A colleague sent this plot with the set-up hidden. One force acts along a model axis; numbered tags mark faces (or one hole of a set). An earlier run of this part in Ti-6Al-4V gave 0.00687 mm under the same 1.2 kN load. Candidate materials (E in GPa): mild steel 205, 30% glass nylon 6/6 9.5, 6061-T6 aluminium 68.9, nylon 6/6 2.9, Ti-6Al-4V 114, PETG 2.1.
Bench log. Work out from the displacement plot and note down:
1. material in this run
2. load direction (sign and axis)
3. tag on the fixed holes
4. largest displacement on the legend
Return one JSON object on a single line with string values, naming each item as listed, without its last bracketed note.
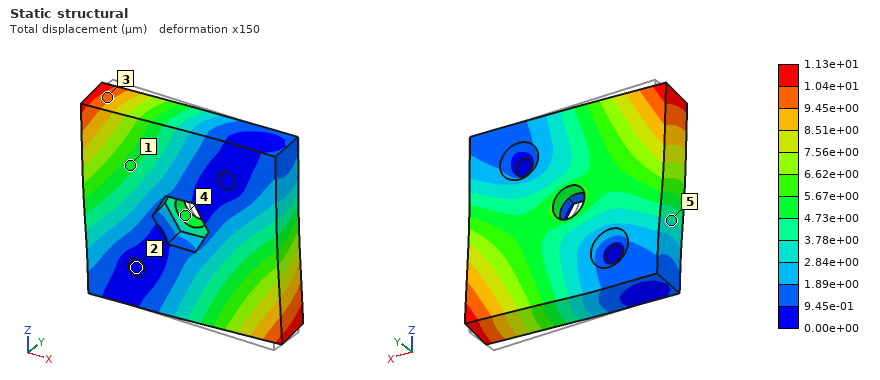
{"material in this run": "6061-T6 aluminium", "load direction": "-X", "tag on the fixed holes": "2", "largest displacement on the legend": "1.13e+01 µm"}
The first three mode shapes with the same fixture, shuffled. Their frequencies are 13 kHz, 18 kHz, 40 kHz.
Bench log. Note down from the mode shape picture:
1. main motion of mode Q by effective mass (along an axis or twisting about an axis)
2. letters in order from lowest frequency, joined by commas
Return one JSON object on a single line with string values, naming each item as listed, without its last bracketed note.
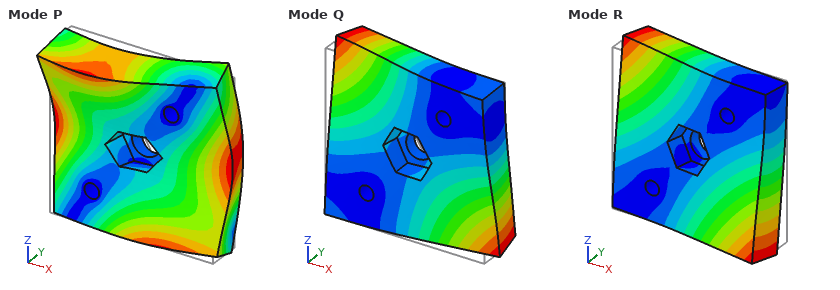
{"main motion of mode Q by effective mass": "along Y", "letters in order from lowest frequency, joined by commas": "R, Q, P"}
